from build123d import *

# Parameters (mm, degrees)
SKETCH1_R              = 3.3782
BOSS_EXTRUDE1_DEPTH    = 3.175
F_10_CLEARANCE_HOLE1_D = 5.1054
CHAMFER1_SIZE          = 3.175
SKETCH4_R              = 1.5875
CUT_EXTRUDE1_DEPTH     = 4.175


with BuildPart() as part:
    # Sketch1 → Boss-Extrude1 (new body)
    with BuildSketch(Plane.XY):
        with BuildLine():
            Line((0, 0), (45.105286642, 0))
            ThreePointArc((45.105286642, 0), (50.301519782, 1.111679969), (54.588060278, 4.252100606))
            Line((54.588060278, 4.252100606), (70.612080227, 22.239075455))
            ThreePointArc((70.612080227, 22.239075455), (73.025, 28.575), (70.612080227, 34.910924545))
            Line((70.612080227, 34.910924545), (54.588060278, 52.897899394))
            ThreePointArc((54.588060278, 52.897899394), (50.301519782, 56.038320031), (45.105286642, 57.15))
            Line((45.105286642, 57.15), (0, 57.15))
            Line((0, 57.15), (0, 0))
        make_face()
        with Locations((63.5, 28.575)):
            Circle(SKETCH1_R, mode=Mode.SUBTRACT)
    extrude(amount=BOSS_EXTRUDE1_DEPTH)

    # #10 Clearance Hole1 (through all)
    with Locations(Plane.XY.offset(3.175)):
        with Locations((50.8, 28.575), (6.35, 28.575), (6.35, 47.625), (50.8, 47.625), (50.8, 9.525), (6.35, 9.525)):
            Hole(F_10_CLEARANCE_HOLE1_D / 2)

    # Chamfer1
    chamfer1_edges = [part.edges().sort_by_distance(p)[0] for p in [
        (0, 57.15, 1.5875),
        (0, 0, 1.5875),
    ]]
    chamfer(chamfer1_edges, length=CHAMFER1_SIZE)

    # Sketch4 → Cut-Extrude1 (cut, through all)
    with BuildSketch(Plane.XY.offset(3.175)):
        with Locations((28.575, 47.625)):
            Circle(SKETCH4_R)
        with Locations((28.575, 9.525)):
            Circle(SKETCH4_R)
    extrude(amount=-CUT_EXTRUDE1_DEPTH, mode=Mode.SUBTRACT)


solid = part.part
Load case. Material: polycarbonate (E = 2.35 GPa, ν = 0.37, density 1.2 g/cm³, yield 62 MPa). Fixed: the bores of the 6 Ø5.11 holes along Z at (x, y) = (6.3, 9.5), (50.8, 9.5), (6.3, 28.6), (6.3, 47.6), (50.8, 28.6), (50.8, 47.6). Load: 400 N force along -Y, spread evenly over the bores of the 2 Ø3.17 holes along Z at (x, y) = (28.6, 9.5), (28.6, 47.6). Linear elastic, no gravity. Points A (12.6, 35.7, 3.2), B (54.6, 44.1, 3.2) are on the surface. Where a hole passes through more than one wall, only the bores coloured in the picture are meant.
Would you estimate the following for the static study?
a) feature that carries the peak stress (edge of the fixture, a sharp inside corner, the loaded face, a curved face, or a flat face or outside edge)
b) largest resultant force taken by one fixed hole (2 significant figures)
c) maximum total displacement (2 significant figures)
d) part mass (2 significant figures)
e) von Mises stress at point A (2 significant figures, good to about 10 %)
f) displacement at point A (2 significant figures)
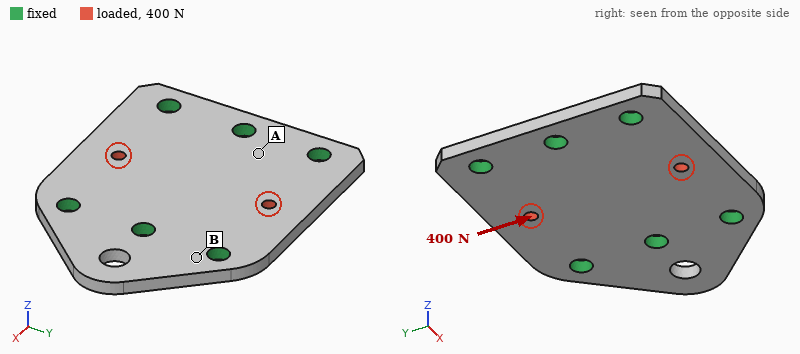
the loaded face
85 N
45 µm
13 g
2.6 MPa
8.7 µm
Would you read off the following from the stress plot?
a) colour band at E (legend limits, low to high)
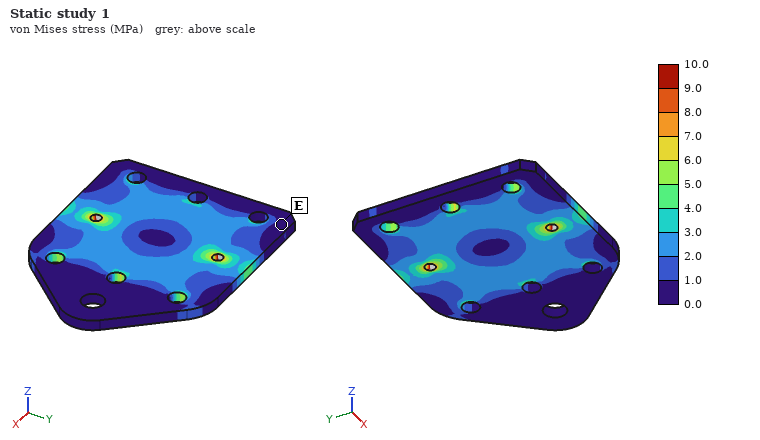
0.0 to 1.0 MPa
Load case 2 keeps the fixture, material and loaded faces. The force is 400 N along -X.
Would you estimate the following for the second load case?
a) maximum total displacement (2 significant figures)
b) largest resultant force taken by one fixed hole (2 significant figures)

24 µm
77 N
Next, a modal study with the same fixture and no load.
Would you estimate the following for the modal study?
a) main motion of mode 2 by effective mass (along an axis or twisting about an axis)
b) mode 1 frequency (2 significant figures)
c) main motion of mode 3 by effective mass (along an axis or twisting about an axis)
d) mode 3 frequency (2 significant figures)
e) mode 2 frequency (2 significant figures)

along Z
2300 Hz
twisting about X
2700 Hz
2500 Hz
